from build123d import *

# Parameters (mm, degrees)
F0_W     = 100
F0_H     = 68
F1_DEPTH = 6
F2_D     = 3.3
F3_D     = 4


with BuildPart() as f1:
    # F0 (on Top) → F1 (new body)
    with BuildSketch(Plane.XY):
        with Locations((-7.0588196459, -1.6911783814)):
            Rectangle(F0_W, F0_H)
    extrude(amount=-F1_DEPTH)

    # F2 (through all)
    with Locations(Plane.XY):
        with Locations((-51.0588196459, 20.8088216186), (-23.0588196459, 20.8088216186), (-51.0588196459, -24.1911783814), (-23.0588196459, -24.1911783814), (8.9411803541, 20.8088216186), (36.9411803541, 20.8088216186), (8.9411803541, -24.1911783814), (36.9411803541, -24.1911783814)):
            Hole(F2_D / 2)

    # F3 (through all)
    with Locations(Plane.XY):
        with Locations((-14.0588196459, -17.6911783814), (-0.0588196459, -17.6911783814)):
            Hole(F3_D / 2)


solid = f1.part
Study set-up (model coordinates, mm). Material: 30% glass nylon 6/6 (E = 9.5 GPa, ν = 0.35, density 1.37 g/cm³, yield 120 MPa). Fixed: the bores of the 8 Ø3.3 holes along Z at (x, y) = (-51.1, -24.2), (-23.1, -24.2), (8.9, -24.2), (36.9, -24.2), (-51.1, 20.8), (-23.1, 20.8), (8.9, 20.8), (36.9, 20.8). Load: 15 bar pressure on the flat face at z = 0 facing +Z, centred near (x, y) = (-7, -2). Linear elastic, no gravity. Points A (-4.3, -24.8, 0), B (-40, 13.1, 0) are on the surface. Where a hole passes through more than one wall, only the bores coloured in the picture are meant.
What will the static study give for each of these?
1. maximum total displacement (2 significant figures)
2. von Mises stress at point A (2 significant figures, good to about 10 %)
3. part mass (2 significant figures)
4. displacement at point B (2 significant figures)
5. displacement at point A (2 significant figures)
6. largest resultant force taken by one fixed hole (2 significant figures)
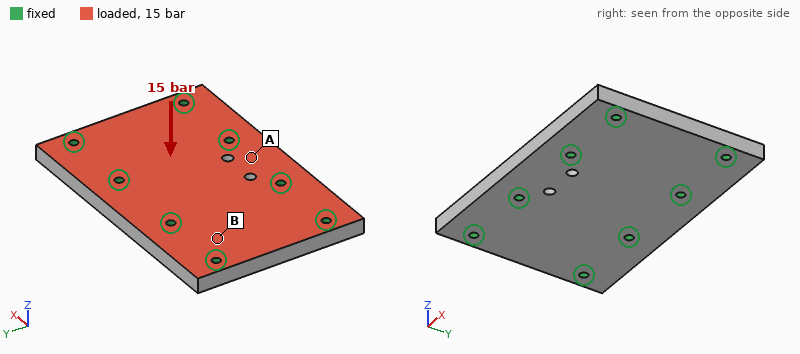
0.16 mm
16 MPa
55 g
0.079 mm
0.051 mm
1.5 kN
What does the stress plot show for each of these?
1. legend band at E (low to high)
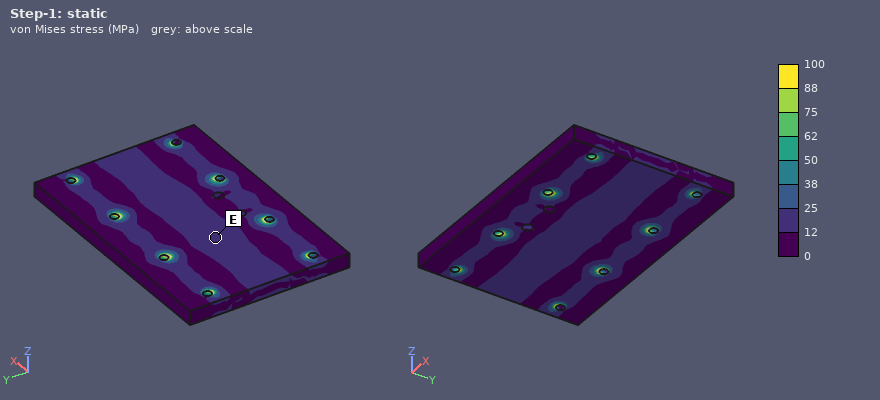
12 to 25 MPa
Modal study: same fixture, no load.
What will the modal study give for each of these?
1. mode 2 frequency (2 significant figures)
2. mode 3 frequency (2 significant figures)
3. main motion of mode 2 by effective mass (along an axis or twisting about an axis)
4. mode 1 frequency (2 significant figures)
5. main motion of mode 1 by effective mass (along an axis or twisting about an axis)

6700 Hz
7700 Hz
twisting about Y
6000 Hz
along Z
